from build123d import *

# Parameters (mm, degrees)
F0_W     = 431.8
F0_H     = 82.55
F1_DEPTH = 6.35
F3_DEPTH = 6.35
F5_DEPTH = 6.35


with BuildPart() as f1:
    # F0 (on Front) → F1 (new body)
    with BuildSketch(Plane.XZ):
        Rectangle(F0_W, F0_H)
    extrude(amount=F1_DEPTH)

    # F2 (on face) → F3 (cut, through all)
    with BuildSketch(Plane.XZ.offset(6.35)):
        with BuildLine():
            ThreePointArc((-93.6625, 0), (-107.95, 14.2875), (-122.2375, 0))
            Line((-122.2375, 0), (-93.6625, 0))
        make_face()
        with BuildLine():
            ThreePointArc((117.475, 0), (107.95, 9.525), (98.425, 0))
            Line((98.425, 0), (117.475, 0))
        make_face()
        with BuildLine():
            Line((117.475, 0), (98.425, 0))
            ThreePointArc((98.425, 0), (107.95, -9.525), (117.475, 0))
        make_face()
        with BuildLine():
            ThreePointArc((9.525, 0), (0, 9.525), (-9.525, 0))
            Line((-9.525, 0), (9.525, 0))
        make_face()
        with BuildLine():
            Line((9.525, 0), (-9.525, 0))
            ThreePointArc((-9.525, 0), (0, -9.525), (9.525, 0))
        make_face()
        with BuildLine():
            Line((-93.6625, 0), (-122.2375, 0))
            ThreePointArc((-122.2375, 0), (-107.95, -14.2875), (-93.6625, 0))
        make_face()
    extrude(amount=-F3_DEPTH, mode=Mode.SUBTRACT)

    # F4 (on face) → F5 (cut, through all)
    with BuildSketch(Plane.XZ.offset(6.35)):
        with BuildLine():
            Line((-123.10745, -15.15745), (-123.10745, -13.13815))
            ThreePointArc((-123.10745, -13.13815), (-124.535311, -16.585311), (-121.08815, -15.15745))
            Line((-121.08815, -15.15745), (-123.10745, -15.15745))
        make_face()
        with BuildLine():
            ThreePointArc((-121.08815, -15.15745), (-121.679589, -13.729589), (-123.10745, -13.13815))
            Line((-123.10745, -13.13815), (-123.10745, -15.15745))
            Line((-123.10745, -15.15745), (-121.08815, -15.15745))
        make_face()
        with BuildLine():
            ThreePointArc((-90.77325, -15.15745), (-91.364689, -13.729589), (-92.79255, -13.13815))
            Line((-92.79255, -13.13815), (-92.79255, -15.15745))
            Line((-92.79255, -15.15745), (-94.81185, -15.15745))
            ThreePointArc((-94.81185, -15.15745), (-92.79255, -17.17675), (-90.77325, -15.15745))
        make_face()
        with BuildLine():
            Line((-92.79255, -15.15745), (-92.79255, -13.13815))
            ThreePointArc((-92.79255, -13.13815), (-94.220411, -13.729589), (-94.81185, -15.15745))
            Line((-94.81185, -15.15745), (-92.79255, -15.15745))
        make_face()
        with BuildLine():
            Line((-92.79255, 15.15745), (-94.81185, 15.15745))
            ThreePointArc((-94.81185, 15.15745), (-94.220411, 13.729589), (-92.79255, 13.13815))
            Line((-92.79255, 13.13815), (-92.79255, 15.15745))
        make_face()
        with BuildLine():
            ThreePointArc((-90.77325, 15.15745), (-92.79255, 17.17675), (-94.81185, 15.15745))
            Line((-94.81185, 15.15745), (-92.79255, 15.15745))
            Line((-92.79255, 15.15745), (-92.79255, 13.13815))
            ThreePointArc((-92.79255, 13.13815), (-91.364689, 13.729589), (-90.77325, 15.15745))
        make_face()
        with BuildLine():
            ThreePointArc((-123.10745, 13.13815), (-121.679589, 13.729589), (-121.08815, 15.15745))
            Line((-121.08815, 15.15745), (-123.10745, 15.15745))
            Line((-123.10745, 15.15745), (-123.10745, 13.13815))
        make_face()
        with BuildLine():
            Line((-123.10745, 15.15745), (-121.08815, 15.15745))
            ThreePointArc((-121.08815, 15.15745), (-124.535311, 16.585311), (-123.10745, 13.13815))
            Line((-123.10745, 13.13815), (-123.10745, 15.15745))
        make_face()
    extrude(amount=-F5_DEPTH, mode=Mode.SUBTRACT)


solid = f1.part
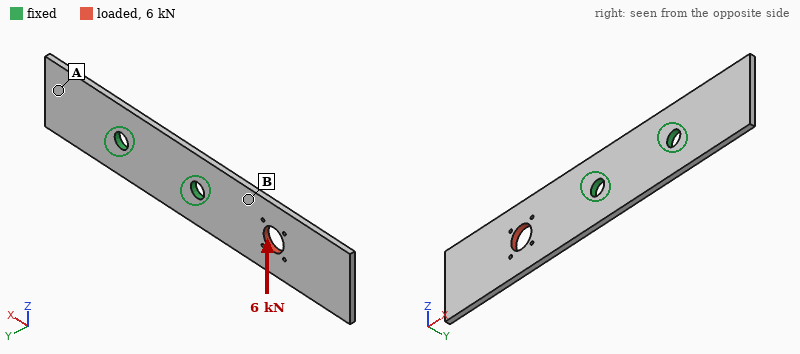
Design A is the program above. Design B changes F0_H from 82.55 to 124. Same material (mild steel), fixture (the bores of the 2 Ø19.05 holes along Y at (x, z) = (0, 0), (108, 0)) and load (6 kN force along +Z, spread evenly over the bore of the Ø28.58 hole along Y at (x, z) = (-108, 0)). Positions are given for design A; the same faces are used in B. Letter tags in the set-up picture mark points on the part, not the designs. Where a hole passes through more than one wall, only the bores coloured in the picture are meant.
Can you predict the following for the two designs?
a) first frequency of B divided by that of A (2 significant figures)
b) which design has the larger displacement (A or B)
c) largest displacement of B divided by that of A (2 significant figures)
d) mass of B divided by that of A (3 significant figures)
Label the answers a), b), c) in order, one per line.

a) 0.98
b) A
c) 0.44
d) 1.52
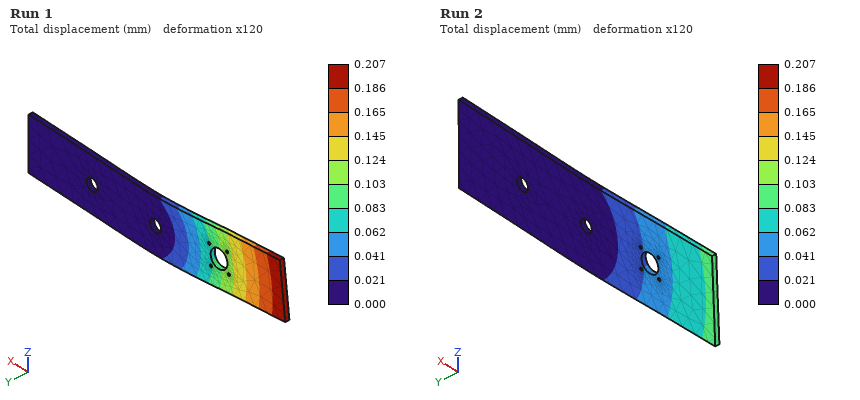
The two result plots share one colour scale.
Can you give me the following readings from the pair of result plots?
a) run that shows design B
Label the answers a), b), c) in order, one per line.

a) Run 2
